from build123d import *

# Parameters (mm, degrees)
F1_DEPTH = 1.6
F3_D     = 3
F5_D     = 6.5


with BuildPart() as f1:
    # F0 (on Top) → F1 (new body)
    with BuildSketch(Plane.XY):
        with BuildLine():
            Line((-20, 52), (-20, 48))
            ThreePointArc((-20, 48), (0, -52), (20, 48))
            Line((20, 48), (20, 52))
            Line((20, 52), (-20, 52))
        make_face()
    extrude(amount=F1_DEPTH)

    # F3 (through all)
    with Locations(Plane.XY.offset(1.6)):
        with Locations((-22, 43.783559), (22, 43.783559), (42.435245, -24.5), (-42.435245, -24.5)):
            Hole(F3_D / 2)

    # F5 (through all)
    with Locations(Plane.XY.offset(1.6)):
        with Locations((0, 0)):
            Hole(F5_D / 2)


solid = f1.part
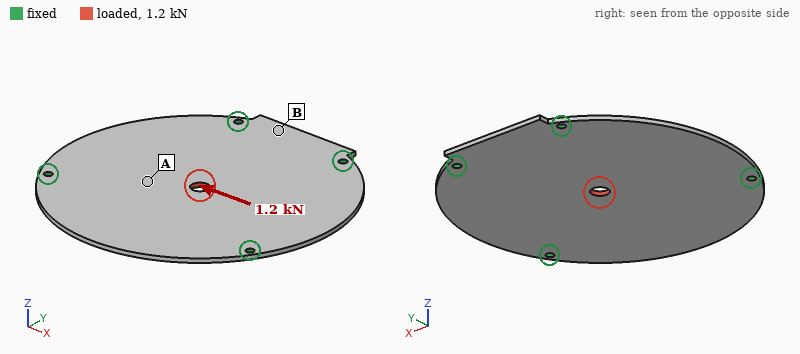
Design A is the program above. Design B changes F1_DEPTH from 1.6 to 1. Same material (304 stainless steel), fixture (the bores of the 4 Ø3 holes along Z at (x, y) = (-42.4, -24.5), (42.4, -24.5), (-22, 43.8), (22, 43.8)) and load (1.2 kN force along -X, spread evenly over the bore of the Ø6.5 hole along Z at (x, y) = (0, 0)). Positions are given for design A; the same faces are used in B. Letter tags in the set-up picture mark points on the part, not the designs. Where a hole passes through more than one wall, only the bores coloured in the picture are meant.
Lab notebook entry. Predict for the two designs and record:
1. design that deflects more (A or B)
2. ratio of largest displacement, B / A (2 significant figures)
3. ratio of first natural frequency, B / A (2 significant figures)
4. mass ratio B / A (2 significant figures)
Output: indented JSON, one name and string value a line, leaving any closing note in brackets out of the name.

{
  "design that deflects more": "B",
  "ratio of largest displacement, B / A": "1.6",
  "ratio of first natural frequency, B / A": "0.63",
  "mass ratio B / A": "0.62"
}
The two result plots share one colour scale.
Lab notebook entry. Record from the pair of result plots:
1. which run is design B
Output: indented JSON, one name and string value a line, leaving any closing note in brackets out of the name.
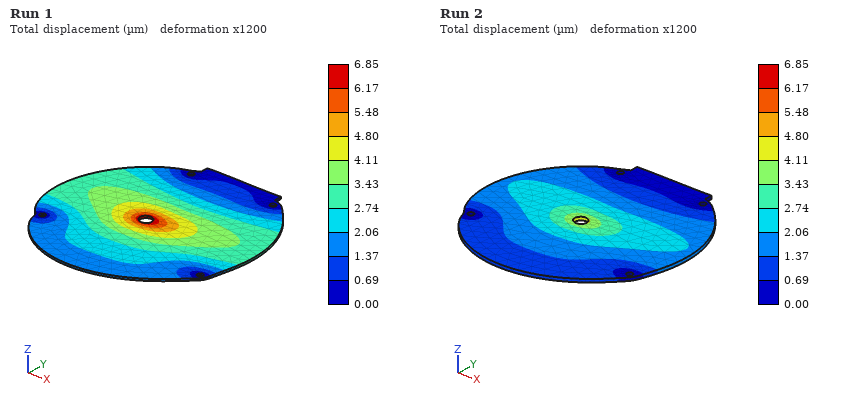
{
  "which run is design B": "Run 1"
}
